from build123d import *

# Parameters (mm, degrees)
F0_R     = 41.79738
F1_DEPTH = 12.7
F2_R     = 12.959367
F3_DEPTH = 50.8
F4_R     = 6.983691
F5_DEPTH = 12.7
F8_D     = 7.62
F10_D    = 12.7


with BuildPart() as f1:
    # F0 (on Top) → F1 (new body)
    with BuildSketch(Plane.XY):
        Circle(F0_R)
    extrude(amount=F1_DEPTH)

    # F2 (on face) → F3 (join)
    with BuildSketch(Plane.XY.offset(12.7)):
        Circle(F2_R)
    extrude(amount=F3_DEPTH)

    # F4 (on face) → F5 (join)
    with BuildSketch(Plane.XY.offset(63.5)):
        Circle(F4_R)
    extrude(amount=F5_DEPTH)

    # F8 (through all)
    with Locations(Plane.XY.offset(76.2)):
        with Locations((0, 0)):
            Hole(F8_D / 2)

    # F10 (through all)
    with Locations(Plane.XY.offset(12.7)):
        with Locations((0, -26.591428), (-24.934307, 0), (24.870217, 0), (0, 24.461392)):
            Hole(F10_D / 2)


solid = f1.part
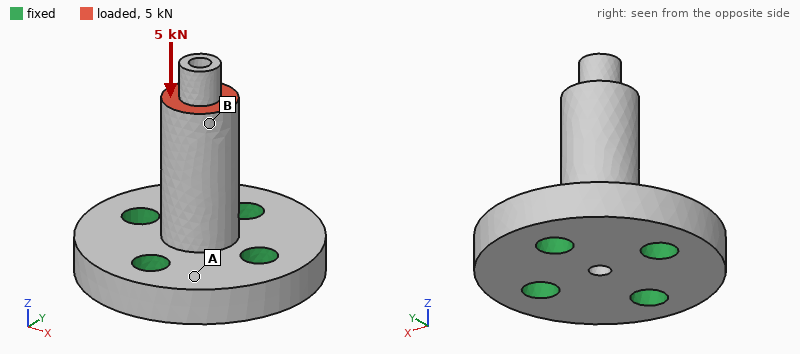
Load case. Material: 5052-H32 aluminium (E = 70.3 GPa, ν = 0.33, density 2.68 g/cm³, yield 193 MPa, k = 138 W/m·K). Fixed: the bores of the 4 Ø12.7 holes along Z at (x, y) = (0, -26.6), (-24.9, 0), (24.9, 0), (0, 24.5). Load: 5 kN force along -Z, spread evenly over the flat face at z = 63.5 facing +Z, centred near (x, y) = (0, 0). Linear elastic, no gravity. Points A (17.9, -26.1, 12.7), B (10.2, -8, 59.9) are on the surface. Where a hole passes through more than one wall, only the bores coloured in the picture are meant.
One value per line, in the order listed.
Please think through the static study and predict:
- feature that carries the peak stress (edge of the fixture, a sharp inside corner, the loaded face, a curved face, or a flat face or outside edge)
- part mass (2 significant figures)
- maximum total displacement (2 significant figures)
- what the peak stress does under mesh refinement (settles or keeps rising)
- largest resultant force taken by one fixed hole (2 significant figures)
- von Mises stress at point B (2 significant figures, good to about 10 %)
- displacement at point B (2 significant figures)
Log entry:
edge of the fixture
240 g
11 µm
keeps rising
1.4 kN
13 MPa
10 µm
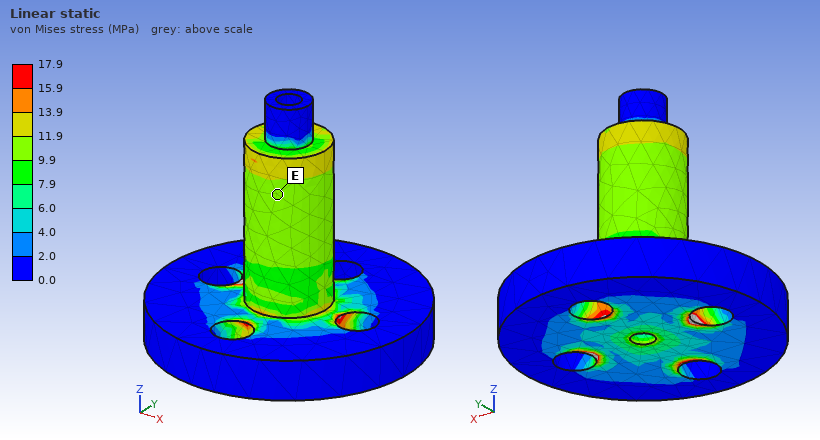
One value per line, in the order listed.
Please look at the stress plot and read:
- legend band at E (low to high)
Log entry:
9.9 to 11.9 MPa
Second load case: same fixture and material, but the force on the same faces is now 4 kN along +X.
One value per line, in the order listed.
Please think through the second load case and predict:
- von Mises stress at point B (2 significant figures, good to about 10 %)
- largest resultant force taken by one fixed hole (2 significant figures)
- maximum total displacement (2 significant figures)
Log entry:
16 MPa
5.9 kN
0.24 mm
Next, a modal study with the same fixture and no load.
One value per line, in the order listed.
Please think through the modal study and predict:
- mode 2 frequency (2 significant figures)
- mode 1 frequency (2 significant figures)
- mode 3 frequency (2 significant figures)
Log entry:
4700 Hz
4700 Hz
14 kHz
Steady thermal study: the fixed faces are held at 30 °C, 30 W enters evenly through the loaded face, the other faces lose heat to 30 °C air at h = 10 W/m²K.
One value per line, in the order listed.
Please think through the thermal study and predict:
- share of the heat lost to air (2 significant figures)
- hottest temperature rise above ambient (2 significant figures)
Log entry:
3.5 %
26 K
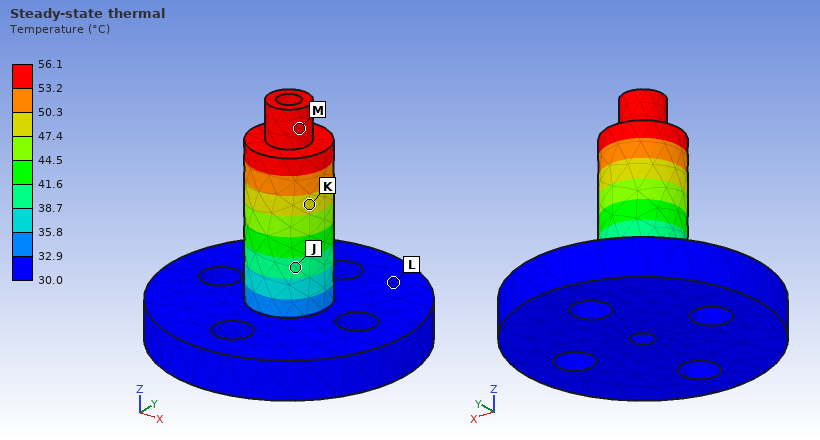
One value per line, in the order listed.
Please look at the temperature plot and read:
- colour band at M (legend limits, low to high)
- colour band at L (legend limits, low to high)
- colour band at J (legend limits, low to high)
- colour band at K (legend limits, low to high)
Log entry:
53.2 to 56.1 °C
30.0 to 32.9 °C
38.7 to 41.6 °C
47.4 to 50.3 °C
